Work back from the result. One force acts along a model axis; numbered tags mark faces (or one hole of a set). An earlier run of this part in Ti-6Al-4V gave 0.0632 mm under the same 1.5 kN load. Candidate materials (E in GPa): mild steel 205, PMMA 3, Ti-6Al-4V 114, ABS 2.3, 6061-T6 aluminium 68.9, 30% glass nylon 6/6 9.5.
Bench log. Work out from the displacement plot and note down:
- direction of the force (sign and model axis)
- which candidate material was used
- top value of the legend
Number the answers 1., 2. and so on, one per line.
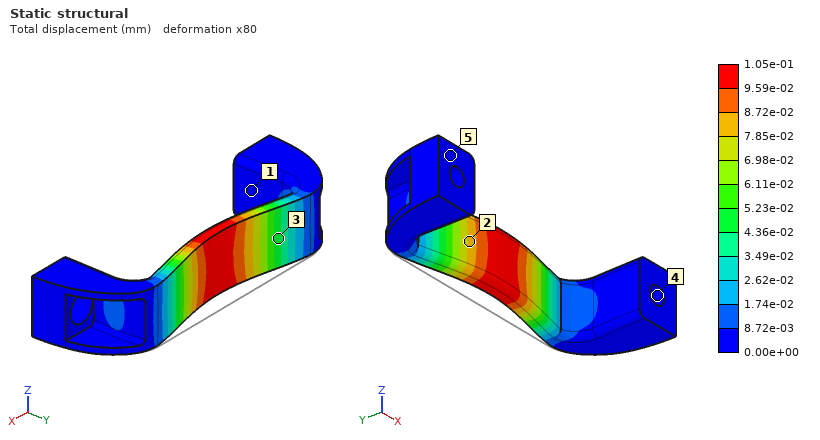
1. -Y
2. 6061-T6 aluminium
3. 1.05e-01 mm
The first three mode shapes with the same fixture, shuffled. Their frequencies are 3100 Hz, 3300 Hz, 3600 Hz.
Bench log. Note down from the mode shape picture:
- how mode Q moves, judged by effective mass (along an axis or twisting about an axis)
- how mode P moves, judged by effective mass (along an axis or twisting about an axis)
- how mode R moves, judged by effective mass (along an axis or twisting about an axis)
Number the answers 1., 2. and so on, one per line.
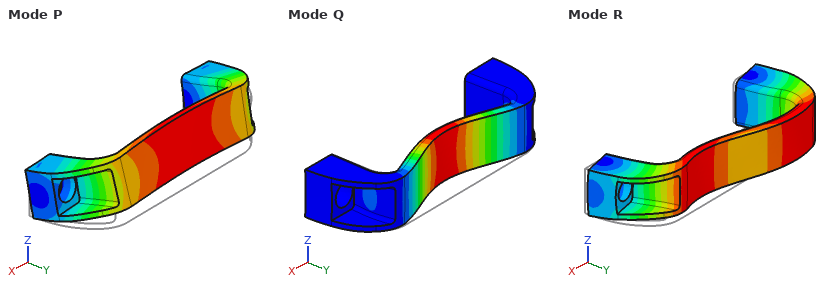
1. along Y
2. along Z
3. along X
